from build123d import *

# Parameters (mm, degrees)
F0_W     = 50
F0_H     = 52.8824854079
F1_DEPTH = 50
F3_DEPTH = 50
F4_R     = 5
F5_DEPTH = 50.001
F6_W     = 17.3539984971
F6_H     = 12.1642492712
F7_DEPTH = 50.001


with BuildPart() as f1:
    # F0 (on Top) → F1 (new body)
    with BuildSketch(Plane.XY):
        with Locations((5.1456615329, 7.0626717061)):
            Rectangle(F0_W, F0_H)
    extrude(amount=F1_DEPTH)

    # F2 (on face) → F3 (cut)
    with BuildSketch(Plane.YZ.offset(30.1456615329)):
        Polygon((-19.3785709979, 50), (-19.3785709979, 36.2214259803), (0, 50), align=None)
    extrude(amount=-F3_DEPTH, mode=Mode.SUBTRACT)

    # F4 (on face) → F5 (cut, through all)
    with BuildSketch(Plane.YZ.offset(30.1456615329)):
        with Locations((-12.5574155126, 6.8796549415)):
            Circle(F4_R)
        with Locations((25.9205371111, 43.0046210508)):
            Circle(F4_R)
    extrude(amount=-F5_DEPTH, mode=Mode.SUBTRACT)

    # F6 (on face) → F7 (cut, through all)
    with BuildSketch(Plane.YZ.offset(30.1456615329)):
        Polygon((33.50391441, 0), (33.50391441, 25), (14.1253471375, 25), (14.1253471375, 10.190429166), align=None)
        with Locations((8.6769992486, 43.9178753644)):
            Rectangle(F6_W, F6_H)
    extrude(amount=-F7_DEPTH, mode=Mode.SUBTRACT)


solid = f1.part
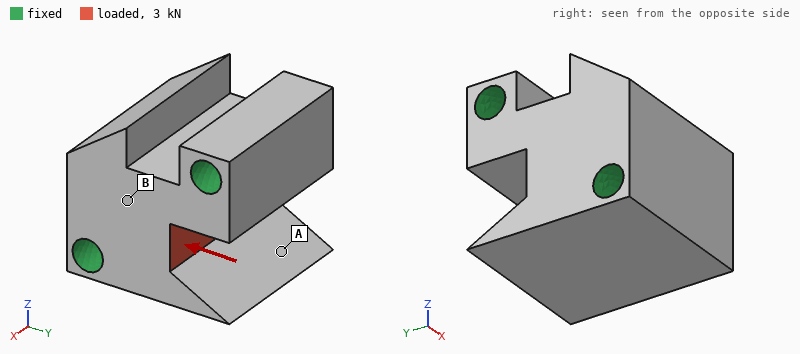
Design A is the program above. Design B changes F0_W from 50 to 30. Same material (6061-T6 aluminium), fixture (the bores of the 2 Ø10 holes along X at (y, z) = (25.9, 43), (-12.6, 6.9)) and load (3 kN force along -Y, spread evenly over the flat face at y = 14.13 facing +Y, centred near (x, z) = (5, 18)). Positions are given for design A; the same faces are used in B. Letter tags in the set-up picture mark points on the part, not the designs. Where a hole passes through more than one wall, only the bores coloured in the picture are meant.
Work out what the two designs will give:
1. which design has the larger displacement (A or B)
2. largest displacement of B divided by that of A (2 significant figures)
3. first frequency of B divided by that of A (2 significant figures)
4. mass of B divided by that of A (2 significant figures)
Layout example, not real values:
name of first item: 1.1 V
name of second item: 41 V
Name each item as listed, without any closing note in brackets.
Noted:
which design has the larger displacement: B
largest displacement of B divided by that of A: 1.7
first frequency of B divided by that of A: 0.99
mass of B divided by that of A: 0.60
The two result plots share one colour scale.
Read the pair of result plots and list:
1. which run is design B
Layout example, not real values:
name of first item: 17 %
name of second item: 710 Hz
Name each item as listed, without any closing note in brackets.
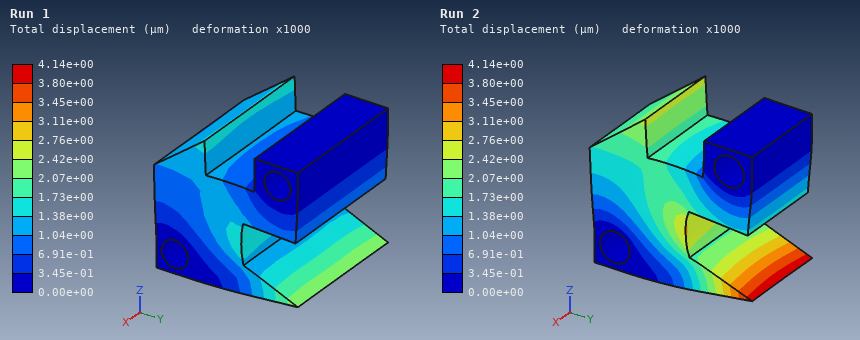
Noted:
which run is design B: Run 2
